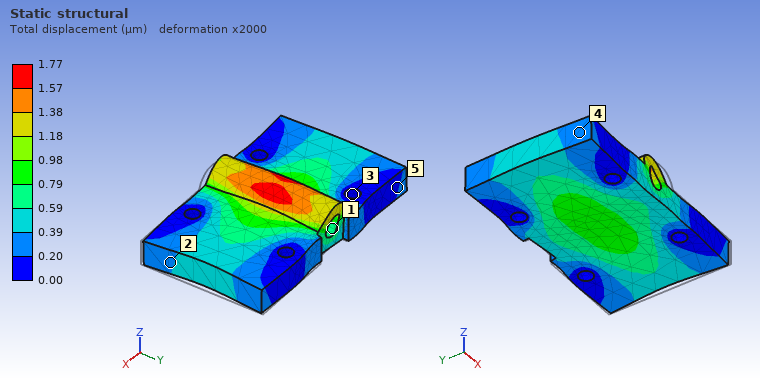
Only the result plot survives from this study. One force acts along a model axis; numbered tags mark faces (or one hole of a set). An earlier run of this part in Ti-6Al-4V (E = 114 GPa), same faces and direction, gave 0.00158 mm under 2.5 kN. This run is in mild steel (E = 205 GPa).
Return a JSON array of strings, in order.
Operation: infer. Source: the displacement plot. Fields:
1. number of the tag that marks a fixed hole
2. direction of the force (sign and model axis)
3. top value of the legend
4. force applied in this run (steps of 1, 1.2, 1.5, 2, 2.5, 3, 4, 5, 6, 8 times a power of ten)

["3", "-X", "1.77 µm", "5 kN"]
